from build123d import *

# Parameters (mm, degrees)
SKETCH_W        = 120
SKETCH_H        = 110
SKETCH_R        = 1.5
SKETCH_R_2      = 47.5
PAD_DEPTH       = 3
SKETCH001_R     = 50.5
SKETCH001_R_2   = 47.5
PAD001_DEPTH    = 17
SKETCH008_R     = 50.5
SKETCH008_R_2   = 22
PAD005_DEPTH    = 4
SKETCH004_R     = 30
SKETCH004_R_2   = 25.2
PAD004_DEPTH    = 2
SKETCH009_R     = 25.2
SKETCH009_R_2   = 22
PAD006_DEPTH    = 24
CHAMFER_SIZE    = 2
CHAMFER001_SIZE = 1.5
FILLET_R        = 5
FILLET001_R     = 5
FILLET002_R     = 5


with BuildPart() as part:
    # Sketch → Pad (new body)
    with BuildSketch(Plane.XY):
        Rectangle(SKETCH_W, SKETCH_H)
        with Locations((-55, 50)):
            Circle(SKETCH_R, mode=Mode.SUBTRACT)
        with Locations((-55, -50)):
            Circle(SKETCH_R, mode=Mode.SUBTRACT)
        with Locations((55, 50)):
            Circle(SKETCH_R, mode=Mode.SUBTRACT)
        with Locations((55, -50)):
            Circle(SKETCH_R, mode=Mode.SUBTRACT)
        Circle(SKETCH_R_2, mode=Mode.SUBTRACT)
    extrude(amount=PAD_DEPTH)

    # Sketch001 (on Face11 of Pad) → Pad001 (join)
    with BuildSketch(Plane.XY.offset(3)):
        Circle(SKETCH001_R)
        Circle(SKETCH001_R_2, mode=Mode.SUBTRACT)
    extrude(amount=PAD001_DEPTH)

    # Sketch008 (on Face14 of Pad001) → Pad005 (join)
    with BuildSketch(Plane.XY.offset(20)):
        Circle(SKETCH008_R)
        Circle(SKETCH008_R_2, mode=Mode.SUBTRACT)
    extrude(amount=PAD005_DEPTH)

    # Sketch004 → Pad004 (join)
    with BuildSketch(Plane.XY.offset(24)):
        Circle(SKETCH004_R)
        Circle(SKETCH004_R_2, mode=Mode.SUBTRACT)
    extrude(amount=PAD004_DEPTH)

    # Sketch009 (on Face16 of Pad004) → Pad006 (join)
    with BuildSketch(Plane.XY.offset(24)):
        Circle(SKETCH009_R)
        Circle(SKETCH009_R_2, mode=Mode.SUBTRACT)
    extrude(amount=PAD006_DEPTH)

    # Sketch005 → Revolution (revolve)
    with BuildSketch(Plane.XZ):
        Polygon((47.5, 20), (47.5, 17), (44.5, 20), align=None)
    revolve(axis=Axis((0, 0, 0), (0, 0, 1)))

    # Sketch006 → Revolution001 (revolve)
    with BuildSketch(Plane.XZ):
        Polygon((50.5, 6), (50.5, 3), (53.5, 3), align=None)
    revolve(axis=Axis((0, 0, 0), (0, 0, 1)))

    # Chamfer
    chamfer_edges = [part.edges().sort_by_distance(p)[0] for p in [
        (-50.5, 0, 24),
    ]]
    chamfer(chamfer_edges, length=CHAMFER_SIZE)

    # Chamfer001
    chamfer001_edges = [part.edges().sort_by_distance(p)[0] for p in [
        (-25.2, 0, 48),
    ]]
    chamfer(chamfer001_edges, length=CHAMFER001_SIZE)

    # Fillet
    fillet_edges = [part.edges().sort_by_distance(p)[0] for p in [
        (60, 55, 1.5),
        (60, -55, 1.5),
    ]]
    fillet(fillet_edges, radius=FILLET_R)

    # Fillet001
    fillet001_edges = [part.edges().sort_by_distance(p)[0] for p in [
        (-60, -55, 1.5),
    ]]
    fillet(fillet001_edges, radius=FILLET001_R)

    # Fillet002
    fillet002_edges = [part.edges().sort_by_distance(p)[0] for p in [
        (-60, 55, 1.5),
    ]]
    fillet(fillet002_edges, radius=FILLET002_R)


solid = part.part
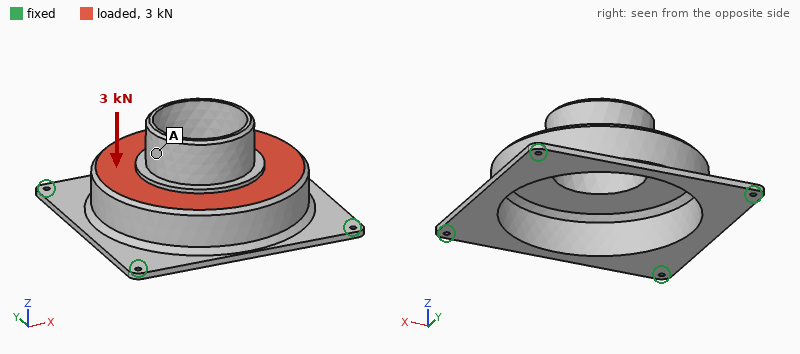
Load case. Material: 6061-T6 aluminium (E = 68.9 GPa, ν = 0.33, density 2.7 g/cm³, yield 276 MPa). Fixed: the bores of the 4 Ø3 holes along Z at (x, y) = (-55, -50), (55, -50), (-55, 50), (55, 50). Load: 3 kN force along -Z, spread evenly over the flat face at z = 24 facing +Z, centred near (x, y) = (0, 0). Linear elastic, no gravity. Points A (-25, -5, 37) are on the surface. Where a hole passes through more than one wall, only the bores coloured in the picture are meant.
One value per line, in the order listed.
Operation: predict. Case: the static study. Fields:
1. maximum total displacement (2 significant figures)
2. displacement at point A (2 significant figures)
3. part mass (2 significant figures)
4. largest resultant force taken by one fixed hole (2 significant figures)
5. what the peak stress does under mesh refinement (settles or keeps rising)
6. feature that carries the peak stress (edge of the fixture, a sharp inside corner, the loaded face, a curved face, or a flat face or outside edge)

0.27 mm
0.27 mm
200 g
1.1 kN
keeps rising
edge of the fixture
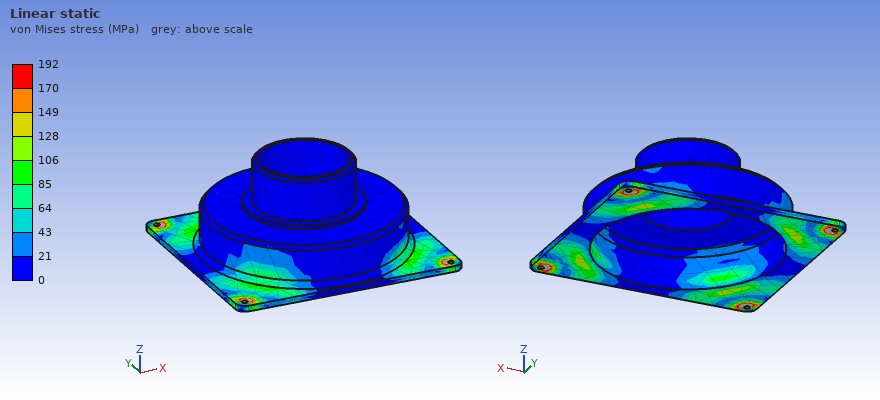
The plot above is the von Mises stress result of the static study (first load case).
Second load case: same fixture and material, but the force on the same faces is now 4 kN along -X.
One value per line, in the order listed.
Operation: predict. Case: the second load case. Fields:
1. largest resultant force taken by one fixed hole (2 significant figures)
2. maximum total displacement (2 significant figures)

1.2 kN
0.17 mm
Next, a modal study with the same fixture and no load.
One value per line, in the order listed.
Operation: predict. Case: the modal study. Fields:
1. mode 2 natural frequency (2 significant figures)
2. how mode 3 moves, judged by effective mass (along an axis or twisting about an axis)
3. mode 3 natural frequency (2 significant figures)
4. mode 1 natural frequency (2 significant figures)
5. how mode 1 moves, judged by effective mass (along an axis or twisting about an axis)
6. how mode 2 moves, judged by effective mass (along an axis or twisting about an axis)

1500 Hz
along X
1700 Hz
1200 Hz
along Z
along Y
